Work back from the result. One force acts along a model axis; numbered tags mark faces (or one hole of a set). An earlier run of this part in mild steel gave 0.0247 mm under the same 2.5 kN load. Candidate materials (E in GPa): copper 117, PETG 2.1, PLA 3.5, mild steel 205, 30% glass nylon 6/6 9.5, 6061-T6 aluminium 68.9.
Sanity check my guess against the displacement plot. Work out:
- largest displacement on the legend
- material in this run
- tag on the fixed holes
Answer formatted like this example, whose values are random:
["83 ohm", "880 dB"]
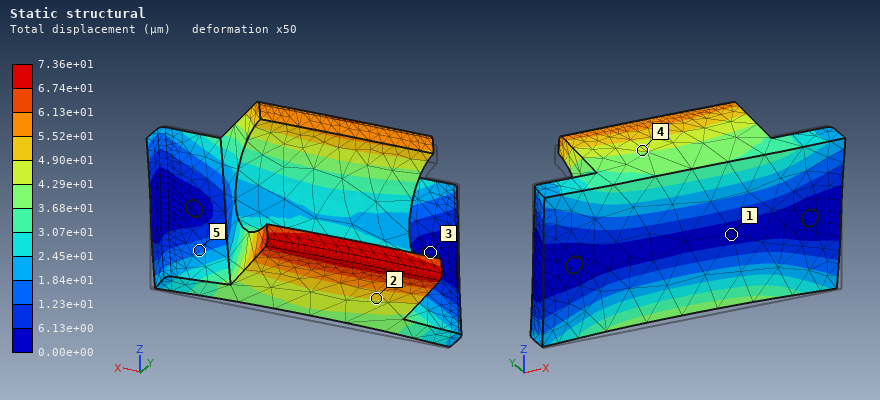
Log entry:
["7.36e+01 µm", "6061-T6 aluminium", "3"]
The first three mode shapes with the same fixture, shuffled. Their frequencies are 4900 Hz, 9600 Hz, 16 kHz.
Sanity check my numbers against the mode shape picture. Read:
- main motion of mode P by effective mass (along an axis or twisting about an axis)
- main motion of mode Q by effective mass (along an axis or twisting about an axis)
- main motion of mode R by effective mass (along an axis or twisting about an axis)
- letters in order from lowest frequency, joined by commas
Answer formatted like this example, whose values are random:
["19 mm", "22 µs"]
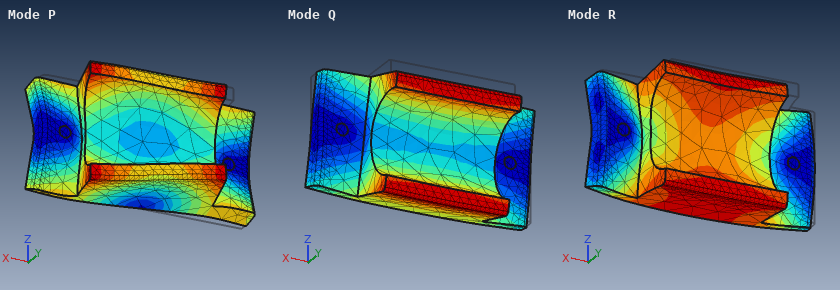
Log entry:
["along X", "along Z", "along Y", "Q, R, P"]
